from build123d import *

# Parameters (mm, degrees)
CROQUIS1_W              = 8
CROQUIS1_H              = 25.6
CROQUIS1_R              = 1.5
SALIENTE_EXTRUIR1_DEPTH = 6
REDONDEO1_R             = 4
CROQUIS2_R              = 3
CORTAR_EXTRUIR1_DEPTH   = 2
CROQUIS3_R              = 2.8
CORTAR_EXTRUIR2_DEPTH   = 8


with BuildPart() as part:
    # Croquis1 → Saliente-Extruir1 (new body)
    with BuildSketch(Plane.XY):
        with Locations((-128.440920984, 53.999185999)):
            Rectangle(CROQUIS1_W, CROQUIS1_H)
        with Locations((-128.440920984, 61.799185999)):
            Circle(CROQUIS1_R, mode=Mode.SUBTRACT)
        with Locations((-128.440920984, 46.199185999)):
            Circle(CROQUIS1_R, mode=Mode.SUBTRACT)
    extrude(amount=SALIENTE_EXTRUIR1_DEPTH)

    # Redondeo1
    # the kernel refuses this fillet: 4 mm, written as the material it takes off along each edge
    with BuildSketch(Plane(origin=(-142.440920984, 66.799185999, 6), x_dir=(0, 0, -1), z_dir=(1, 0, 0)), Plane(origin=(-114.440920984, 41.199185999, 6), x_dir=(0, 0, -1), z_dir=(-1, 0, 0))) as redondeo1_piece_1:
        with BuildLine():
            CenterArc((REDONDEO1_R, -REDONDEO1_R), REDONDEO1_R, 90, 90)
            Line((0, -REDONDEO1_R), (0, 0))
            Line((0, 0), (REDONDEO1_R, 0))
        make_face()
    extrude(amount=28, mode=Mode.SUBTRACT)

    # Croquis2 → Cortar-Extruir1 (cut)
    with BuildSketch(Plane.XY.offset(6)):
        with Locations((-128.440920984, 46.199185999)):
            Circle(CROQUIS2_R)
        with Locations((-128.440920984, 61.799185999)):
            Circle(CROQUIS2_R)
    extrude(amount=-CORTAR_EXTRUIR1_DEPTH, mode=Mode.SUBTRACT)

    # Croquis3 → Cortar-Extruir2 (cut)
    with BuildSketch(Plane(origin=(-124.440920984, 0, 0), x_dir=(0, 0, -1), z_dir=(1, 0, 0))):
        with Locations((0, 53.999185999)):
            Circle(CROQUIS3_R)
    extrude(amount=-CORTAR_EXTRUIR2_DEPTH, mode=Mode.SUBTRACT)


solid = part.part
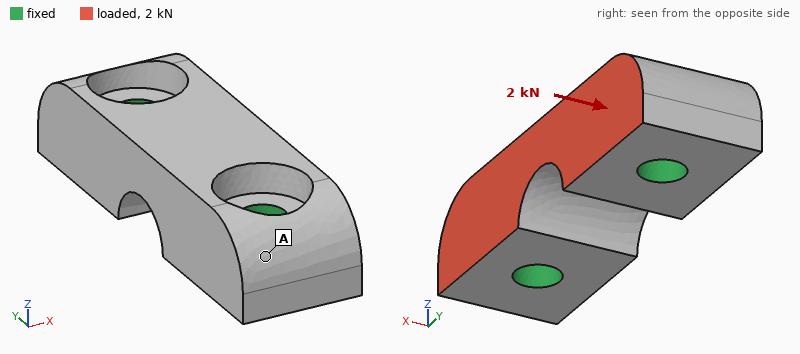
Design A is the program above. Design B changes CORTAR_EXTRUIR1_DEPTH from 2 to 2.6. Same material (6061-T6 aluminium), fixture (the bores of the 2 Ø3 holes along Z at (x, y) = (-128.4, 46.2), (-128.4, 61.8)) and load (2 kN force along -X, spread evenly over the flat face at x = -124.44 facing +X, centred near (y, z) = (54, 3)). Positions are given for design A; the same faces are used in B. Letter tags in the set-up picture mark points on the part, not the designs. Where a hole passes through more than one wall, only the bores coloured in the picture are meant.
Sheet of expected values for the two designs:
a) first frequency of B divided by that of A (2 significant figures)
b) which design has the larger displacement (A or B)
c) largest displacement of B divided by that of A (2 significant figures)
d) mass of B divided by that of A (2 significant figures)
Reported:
0.87
B
1.4
0.97
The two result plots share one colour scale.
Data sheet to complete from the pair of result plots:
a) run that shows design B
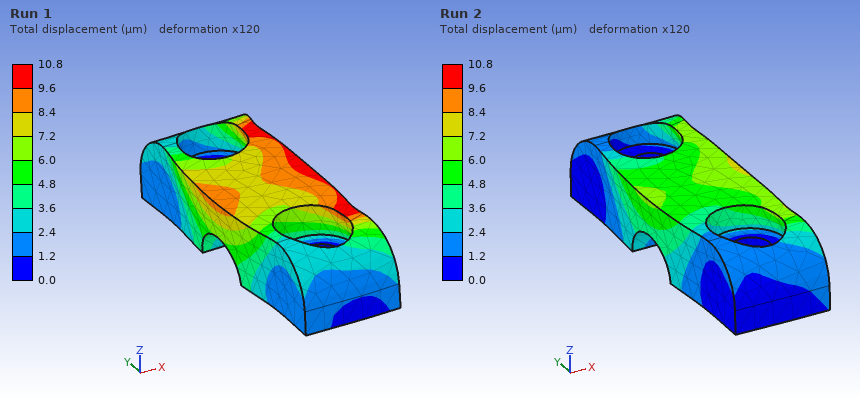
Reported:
Run 1
